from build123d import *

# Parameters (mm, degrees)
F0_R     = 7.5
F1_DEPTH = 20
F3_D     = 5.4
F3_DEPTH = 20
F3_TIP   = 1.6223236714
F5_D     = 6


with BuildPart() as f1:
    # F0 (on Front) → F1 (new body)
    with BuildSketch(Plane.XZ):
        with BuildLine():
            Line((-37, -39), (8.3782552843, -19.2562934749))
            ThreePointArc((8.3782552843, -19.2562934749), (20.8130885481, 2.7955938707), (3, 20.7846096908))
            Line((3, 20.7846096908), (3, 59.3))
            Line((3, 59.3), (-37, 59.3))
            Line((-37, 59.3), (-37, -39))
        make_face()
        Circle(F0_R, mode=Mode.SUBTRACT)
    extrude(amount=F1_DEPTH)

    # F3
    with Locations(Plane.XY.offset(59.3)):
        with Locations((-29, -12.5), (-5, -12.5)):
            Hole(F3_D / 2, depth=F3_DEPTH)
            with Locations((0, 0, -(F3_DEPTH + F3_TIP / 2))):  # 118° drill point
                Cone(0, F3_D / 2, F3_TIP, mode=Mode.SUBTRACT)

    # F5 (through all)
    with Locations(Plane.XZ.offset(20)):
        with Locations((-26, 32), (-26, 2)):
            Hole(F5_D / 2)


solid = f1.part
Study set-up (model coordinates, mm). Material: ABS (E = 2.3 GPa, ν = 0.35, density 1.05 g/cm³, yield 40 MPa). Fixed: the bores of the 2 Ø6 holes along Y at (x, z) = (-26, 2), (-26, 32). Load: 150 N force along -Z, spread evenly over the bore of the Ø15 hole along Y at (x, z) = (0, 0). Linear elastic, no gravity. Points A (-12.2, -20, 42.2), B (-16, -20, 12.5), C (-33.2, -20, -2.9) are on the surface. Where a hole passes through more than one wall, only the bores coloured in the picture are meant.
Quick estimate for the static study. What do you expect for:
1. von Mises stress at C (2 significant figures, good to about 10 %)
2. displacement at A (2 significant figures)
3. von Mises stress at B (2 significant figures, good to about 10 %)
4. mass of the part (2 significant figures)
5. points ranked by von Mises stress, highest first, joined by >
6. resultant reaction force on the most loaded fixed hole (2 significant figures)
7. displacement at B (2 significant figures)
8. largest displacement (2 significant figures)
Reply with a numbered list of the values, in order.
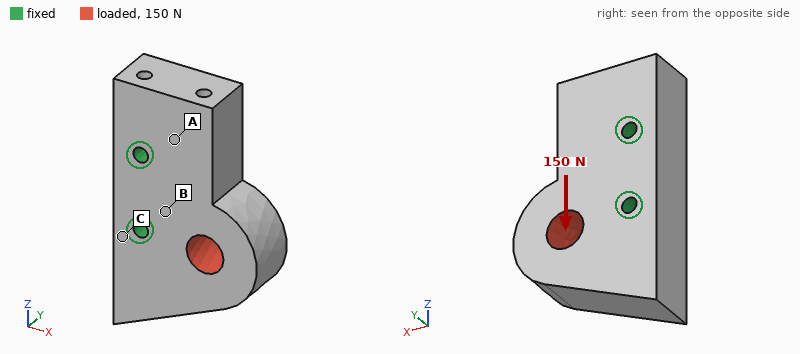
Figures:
1. 0.22 MPa
2. 4.3 µm
3. 0.36 MPa
4. 81 g
5. B > C > A
6. 130 N
7. 2.4 µm
8. 15 µm
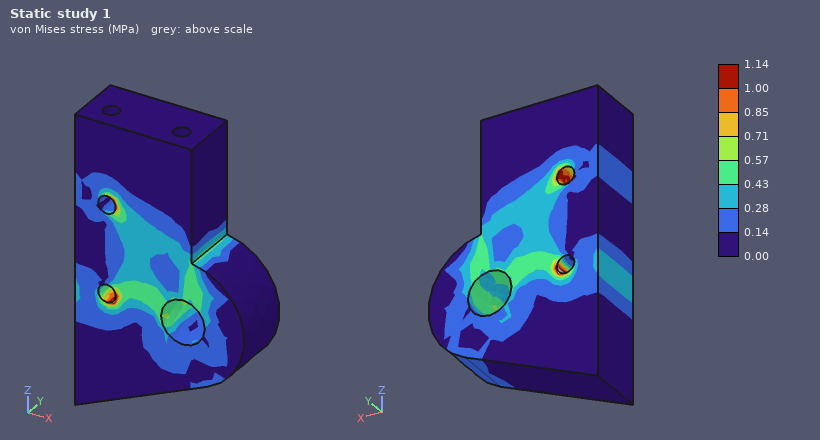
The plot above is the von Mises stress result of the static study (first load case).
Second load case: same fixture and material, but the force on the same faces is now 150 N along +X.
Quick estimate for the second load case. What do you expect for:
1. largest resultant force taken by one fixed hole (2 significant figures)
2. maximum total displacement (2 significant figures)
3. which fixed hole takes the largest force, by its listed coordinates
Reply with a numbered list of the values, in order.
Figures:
1. 150 N
2. 9.6 µm
3. (-26, 2)
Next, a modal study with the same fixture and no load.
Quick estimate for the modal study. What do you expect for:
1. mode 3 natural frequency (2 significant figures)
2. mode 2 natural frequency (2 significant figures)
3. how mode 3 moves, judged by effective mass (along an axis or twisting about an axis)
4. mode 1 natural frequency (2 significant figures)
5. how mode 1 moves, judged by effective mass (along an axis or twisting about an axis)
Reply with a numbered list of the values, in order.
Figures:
1. 2800 Hz
2. 2500 Hz
3. twisting about X
4. 2000 Hz
5. along Y
